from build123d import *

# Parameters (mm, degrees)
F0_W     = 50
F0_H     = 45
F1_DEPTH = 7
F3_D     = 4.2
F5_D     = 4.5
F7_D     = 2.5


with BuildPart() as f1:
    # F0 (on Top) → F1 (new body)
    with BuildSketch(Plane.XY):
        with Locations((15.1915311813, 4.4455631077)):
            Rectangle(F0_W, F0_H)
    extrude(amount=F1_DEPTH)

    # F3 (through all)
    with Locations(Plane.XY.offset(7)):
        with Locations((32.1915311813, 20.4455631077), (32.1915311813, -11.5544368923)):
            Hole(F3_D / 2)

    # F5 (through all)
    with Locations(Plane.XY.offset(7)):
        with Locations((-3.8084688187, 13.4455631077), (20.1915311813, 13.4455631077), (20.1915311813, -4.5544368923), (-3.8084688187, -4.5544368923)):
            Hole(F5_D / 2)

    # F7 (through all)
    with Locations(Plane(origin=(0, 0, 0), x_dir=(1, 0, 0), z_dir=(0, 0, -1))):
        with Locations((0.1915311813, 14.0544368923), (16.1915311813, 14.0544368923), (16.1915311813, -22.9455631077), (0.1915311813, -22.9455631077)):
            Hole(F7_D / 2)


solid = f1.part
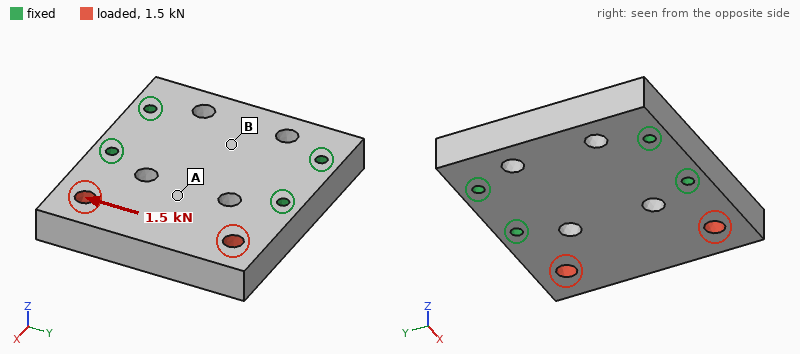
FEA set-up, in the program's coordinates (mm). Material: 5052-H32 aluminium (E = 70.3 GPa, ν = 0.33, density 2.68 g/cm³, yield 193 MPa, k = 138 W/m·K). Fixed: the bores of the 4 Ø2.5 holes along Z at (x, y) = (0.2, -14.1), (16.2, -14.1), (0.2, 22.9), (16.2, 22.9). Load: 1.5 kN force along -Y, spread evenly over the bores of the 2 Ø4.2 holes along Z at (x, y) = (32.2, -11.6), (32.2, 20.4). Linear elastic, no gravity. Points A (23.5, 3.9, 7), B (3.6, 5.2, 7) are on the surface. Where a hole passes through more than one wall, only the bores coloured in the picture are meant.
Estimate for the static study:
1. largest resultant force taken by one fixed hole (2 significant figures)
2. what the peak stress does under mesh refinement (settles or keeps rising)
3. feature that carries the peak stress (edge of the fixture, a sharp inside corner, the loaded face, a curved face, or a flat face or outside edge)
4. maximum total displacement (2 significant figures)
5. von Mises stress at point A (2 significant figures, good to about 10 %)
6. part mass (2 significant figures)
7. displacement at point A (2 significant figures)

870 N
keeps rising
edge of the fixture
6.2 µm
8.7 MPa
40 g
2.8 µm
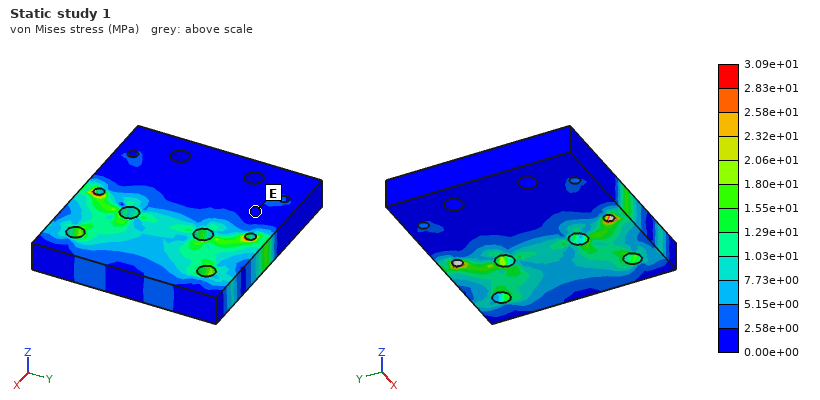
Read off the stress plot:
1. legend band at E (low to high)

0.00e+00 to 2.58e+00 MPa
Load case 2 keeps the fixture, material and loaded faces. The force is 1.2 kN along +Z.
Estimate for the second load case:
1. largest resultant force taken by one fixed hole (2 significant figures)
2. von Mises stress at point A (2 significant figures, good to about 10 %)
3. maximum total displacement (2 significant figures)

820 N
22 MPa
56 µm
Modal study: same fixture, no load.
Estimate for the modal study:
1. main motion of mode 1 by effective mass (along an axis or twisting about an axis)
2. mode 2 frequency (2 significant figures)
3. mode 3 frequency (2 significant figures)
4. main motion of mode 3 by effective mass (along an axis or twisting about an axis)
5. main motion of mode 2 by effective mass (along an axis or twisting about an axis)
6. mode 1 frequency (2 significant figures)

along Z
13 kHz
18 kHz
along Z
twisting about X
7200 Hz
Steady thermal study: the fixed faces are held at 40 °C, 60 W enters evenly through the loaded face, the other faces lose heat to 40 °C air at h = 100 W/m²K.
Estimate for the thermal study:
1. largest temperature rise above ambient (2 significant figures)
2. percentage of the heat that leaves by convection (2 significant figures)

34 K
11 %
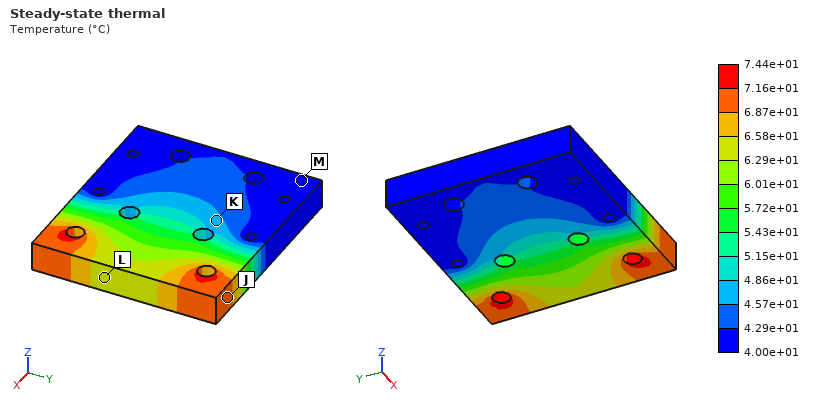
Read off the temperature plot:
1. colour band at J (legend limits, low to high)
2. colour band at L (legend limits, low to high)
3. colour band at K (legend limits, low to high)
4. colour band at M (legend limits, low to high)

6.87e+01 to 7.16e+01 °C
6.29e+01 to 6.58e+01 °C
4.57e+01 to 4.86e+01 °C
4.00e+01 to 4.29e+01 °C
